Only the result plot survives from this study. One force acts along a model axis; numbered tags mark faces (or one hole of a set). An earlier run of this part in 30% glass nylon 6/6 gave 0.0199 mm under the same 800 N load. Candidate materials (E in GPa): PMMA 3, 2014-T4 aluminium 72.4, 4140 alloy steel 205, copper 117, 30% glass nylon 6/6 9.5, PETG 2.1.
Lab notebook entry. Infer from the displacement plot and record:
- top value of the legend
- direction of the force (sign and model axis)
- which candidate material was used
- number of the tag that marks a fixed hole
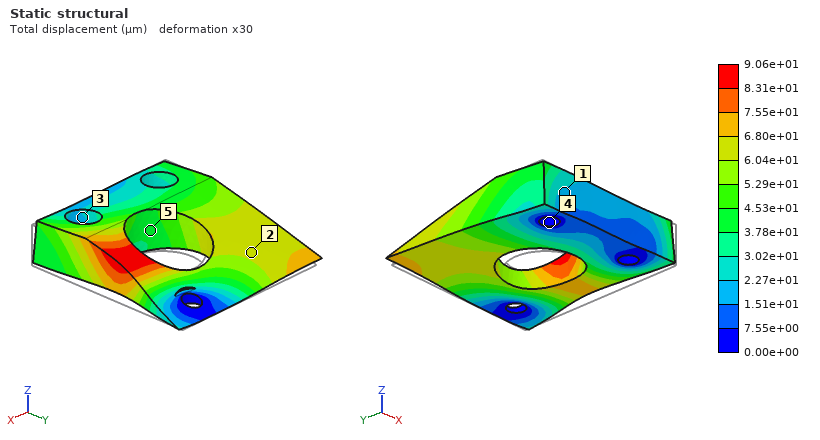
9.06e+01 µm
-X
PETG
4
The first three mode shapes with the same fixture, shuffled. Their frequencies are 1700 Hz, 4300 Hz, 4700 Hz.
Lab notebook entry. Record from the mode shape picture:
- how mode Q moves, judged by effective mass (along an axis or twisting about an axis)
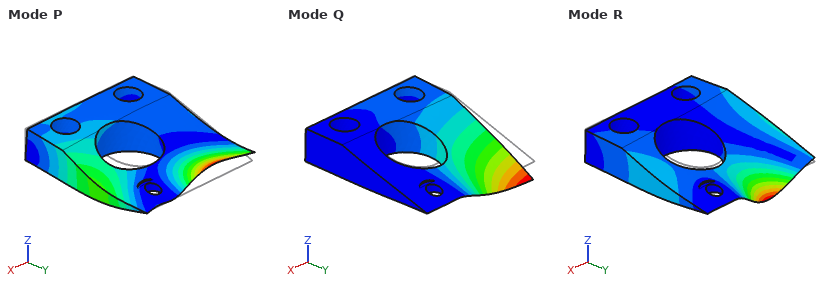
along Z
